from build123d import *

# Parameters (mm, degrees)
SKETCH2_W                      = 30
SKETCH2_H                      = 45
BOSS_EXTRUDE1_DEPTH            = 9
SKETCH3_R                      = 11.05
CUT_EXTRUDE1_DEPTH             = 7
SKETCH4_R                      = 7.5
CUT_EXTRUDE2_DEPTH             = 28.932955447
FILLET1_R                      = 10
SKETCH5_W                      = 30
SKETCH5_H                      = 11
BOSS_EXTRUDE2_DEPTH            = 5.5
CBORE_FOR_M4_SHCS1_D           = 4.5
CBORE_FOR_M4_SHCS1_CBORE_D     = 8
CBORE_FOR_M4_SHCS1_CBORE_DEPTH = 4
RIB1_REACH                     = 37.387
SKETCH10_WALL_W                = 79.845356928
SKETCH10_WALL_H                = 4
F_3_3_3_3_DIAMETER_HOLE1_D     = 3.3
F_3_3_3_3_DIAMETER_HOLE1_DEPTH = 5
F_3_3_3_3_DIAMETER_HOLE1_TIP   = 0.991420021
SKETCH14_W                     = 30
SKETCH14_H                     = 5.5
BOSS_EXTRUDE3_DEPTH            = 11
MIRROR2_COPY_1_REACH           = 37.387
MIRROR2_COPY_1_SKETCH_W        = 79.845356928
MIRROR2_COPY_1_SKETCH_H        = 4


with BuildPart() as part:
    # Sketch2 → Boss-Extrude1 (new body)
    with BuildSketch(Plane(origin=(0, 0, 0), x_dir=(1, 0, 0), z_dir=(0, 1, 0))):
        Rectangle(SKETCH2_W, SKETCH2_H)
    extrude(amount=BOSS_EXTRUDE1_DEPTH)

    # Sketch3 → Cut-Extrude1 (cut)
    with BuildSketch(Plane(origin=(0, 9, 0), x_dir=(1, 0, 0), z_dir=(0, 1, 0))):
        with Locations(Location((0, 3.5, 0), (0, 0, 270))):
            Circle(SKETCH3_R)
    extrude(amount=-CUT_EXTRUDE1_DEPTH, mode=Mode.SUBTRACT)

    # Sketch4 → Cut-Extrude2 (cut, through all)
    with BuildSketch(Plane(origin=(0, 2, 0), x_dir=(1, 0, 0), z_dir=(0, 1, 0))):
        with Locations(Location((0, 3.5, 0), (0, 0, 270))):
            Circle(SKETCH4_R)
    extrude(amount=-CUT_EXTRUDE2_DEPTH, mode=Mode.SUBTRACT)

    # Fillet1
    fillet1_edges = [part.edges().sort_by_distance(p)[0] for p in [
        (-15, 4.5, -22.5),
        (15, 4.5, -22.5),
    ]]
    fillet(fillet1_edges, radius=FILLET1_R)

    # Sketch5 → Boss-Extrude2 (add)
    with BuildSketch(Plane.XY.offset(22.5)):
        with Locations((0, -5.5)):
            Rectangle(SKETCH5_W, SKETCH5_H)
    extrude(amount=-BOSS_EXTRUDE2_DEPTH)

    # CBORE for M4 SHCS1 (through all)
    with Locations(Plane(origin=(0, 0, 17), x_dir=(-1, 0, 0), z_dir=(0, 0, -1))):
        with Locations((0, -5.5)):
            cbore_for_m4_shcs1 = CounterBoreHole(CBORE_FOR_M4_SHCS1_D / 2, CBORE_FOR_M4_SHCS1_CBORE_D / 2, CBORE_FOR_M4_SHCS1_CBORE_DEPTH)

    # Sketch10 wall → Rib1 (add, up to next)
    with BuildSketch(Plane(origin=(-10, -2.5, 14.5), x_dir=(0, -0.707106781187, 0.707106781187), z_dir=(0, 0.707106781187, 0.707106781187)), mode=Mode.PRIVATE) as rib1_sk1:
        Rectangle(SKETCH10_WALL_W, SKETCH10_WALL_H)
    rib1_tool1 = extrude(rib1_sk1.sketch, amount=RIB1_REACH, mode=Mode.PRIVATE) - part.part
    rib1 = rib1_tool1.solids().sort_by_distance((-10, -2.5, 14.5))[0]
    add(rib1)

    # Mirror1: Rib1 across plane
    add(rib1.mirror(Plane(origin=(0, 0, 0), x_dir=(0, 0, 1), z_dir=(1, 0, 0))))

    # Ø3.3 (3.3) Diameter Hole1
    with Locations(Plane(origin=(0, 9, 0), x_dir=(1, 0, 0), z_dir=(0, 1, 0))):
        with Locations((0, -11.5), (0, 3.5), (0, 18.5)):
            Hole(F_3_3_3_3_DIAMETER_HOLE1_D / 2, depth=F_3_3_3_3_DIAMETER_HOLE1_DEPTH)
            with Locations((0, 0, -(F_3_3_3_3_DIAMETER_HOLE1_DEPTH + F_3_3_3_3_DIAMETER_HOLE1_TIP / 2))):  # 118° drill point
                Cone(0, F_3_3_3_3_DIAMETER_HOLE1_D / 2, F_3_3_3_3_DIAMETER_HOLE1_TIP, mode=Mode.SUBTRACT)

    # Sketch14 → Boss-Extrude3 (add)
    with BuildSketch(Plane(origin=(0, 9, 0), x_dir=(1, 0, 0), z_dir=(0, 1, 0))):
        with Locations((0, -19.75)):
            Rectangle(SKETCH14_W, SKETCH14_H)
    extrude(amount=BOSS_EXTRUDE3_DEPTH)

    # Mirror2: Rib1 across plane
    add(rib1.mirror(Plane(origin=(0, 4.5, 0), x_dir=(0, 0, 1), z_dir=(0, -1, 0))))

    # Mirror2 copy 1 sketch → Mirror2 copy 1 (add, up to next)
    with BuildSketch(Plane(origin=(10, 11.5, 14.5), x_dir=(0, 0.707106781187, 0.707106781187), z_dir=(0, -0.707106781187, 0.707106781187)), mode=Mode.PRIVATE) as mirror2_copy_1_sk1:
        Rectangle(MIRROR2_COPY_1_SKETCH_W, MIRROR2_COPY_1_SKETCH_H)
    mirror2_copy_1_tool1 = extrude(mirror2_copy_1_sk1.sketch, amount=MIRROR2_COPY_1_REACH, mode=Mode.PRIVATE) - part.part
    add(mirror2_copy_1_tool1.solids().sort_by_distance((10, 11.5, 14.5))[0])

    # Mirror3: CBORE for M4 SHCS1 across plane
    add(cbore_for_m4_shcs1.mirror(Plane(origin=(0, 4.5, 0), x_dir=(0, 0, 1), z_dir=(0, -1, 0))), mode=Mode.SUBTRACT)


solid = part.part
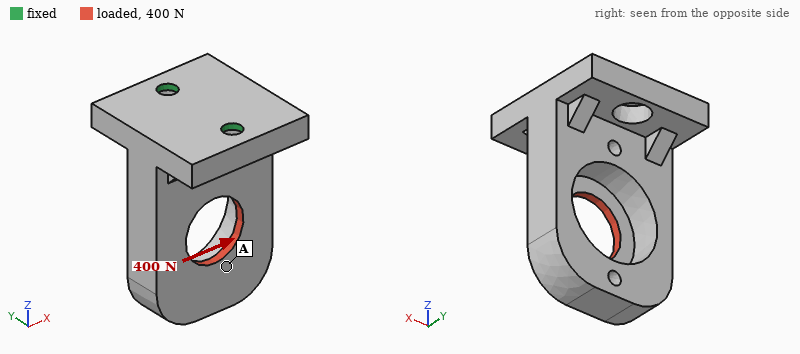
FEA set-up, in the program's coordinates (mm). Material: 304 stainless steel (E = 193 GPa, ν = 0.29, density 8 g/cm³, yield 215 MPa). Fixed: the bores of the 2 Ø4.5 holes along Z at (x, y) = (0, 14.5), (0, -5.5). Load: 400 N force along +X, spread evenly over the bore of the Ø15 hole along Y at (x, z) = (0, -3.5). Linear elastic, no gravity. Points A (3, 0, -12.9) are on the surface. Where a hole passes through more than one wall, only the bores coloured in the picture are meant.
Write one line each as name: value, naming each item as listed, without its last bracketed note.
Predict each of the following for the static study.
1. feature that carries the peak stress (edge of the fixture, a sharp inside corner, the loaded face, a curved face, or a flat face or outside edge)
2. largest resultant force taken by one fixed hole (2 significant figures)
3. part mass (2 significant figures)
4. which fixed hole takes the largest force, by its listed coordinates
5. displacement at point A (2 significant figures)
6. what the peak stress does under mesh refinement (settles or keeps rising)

feature that carries the peak stress: edge of the fixture
largest resultant force taken by one fixed hole: 260 N
part mass: 96 g
which fixed hole takes the largest force, by its listed coordinates: (0, -5.5)
displacement at point A: 78 µm
what the peak stress does under mesh refinement: keeps rising
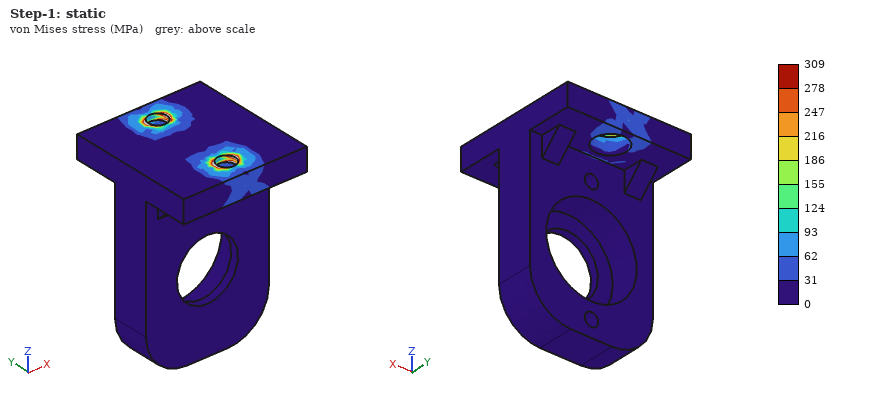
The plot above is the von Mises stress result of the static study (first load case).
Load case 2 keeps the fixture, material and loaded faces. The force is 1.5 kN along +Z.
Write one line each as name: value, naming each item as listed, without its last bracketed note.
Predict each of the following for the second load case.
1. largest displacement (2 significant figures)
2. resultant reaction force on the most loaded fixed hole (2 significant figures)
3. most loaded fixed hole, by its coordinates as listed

largest displacement: 18 µm
resultant reaction force on the most loaded fixed hole: 1.1 kN
most loaded fixed hole, by its coordinates as listed: (0, -5.5)
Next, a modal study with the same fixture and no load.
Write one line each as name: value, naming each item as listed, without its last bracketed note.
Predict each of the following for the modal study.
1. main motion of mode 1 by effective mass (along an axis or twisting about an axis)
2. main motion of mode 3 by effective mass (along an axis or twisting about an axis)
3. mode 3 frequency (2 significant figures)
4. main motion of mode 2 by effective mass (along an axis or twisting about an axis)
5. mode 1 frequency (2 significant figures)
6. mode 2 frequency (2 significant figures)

main motion of mode 1 by effective mass: along X
main motion of mode 3 by effective mass: twisting about Z
mode 3 frequency: 8800 Hz
main motion of mode 2 by effective mass: along Y
mode 1 frequency: 1500 Hz
mode 2 frequency: 3400 Hz
